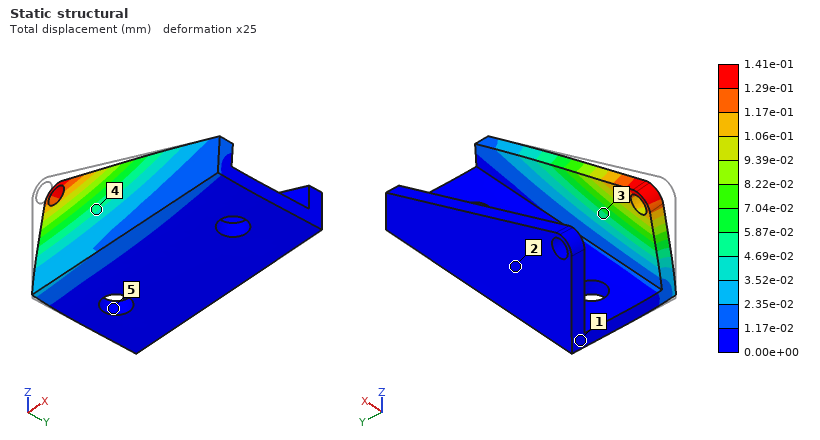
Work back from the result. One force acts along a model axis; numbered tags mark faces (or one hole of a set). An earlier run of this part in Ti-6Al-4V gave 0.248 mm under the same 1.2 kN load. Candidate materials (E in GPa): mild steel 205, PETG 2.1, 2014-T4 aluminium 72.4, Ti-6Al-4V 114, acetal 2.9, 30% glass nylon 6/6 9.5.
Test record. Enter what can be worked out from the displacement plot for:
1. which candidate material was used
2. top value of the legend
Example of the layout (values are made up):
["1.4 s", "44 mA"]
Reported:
["mild steel", "1.41e-01 mm"]
